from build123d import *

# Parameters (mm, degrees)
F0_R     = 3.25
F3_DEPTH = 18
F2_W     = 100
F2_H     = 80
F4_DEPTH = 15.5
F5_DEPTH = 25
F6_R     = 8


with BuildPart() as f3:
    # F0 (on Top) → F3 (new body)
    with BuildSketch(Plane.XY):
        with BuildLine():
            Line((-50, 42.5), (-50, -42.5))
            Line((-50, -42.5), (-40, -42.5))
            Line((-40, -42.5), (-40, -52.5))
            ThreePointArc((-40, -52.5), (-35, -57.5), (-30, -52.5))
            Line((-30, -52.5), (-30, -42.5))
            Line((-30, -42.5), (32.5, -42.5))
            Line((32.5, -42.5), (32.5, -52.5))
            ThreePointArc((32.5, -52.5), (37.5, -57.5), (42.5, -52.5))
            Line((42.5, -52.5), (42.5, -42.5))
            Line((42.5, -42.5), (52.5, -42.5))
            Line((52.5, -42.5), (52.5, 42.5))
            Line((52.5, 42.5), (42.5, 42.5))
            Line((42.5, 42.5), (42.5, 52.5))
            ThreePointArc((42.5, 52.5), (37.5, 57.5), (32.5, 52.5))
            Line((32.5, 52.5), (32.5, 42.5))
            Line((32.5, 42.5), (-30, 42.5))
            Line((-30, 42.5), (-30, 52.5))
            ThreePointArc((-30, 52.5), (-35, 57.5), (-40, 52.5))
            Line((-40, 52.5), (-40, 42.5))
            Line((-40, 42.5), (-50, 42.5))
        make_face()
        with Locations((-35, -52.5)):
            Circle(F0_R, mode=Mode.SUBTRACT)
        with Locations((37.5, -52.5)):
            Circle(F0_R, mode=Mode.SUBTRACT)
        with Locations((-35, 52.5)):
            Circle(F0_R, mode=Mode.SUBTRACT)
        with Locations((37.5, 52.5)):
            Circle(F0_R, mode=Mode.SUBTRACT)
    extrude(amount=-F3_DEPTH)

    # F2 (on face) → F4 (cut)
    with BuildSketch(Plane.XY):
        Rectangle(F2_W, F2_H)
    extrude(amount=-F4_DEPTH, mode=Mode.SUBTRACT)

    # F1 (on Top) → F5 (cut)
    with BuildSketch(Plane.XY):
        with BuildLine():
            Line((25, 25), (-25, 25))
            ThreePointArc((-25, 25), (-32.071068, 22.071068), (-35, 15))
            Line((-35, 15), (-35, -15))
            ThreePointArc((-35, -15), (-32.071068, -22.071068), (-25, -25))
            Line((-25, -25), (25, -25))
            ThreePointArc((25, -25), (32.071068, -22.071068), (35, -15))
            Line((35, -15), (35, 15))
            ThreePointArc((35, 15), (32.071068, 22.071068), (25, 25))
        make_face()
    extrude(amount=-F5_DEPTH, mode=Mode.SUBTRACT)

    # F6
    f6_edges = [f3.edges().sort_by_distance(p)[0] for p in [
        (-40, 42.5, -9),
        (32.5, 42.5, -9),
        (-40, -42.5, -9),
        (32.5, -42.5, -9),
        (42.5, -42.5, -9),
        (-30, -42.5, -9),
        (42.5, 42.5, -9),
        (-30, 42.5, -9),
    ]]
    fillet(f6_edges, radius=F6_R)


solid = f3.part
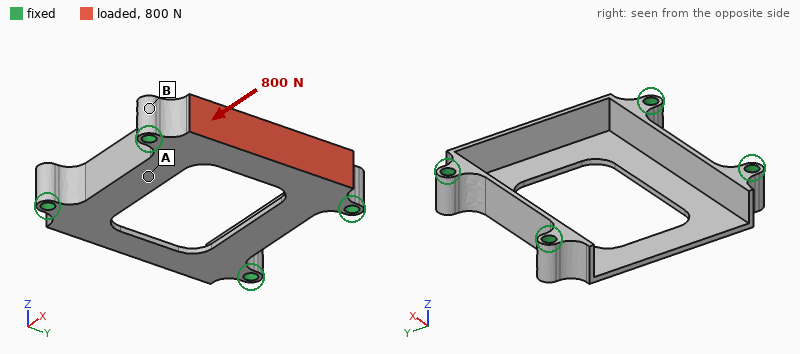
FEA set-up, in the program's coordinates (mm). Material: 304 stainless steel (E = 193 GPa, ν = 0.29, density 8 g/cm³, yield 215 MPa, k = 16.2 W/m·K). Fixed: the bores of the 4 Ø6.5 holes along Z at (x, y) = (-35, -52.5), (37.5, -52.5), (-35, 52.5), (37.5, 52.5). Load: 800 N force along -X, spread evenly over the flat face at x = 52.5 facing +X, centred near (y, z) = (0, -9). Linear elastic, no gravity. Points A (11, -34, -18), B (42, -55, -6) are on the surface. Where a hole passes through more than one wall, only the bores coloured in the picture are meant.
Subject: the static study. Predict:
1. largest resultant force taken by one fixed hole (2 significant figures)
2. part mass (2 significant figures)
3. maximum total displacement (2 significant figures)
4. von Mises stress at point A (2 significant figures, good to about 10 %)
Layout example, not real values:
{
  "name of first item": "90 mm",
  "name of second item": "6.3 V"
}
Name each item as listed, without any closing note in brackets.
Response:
{
  "largest resultant force taken by one fixed hole": "360 N",
  "part mass": "270 g",
  "maximum total displacement": "57 µm",
  "von Mises stress at point A": "8.4 MPa"
}
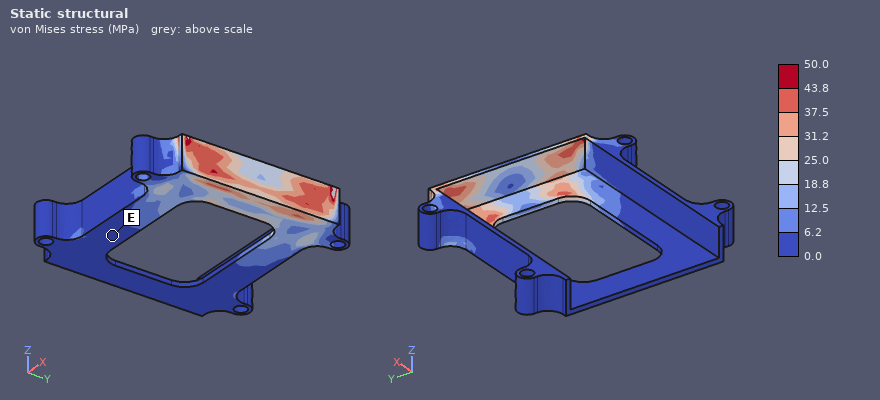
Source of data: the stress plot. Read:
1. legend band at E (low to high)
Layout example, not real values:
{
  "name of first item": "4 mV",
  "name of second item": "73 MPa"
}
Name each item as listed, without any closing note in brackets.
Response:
{
  "legend band at E": "0.0 to 6.2 MPa"
}
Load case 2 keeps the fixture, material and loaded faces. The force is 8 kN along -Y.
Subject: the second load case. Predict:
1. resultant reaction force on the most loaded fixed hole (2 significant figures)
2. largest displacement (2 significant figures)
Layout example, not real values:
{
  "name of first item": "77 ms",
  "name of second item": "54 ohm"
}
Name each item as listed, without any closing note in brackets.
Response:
{
  "resultant reaction force on the most loaded fixed hole": "4.2 kN",
  "largest displacement": "24 µm"
}
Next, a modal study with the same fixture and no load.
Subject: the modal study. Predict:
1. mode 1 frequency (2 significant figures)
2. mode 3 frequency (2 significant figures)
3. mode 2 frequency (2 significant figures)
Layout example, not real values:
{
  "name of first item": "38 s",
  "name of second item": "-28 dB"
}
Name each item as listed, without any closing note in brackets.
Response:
{
  "mode 1 frequency": "2200 Hz",
  "mode 3 frequency": "4800 Hz",
  "mode 2 frequency": "3800 Hz"
}
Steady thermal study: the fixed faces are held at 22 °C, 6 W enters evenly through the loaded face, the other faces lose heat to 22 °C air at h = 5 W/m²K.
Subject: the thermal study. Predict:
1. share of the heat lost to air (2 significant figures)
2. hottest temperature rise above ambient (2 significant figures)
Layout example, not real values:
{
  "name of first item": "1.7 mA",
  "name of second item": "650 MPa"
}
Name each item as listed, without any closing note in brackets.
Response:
{
  "share of the heat lost to air": "16 %",
  "hottest temperature rise above ambient": "53 K"
}
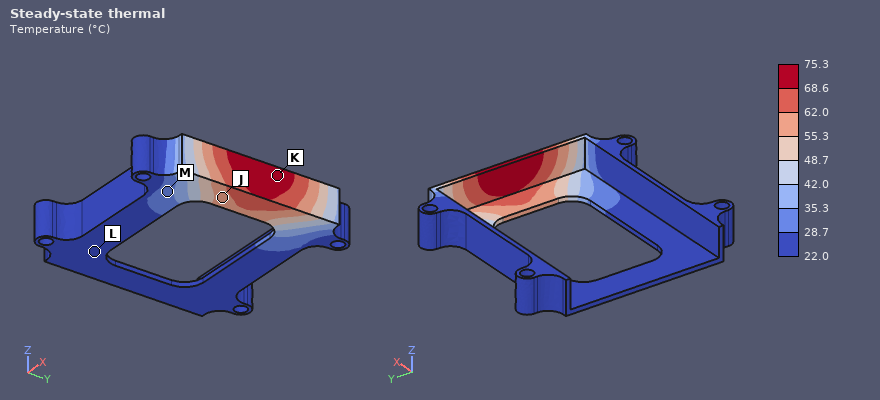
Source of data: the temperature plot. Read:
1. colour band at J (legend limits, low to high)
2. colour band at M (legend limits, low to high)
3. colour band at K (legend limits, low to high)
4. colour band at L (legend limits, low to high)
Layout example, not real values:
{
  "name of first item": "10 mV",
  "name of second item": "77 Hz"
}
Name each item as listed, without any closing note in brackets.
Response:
{
  "colour band at J": "55.3 to 62.0 °C",
  "colour band at M": "28.7 to 35.3 °C",
  "colour band at K": "68.6 to 75.3 °C",
  "colour band at L": "22.0 to 28.7 °C"
}
